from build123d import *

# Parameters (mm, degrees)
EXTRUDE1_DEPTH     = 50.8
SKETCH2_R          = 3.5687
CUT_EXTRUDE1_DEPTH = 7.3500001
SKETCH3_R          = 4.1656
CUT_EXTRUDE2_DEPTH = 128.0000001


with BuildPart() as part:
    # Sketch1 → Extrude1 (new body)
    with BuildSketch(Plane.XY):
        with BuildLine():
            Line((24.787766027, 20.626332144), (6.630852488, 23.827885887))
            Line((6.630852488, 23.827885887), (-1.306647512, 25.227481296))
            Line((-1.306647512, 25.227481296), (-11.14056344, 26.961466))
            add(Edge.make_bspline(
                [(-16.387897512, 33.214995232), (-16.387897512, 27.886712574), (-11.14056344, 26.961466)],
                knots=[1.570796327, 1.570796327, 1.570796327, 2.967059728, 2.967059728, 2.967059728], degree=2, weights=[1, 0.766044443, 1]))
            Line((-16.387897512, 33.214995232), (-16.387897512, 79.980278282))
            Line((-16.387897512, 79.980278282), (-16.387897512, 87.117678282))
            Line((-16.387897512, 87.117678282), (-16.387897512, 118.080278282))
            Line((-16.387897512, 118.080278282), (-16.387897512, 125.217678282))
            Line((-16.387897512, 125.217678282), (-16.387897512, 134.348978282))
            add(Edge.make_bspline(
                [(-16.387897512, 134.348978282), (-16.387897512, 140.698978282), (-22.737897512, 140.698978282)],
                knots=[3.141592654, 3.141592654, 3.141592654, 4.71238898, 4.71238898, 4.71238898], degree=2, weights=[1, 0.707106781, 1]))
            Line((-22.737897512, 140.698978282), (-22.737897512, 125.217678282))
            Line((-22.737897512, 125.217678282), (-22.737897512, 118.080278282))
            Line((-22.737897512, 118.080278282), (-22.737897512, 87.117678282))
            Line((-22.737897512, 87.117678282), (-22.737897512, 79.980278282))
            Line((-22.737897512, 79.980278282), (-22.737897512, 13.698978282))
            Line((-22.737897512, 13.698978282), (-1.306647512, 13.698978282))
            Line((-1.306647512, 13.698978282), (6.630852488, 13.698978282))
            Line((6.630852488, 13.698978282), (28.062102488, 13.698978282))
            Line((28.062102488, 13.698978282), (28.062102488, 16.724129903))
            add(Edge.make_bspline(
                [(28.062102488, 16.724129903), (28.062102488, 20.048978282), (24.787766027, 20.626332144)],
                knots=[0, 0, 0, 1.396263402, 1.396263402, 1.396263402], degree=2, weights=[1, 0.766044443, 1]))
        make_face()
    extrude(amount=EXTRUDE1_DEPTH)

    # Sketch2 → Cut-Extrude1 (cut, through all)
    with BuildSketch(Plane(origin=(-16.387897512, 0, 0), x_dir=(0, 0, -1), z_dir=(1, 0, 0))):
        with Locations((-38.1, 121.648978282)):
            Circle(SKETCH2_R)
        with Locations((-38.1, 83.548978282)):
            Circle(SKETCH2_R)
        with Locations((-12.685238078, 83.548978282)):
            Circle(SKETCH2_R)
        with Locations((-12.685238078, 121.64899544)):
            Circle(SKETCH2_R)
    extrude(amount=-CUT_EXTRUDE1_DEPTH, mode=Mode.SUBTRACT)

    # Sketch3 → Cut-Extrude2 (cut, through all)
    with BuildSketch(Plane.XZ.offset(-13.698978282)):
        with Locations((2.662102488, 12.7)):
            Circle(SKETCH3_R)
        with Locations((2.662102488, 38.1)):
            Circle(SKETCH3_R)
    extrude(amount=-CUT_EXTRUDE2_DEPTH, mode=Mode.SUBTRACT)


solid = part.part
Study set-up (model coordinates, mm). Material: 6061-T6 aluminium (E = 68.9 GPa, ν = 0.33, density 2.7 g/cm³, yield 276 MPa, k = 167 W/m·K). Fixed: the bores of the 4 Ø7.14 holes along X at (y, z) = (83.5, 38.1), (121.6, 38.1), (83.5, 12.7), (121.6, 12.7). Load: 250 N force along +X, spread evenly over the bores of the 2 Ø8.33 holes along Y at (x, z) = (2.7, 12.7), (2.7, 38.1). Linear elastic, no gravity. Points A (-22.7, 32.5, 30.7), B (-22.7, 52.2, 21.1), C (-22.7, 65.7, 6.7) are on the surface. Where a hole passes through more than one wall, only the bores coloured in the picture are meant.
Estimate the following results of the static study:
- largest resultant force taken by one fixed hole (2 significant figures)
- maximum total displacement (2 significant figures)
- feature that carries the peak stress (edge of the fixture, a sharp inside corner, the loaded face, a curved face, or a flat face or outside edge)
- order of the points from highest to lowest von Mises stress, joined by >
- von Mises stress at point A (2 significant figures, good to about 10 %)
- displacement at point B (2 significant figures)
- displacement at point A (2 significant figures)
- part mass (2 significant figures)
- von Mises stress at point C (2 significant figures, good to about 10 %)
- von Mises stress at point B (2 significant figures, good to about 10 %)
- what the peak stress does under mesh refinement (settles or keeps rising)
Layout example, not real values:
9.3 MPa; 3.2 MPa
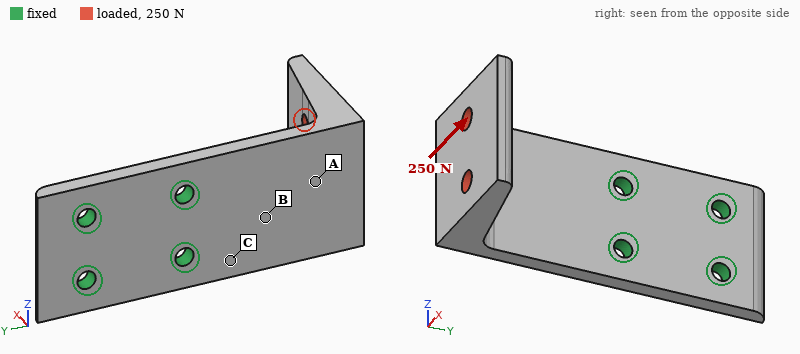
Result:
150 N; 0.43 mm; edge of the fixture; C > B > A; 9.2 MPa; 0.081 mm; 0.19 mm; 170 g; 33 MPa; 22 MPa; keeps rising
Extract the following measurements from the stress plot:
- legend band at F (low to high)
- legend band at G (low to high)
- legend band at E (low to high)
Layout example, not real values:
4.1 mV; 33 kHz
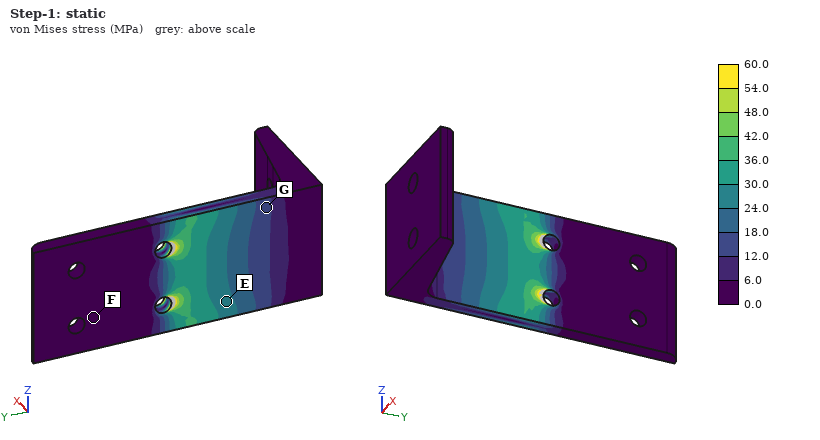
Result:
0.0 to 6.0 MPa; 12.0 to 18.0 MPa; 24.0 to 30.0 MPa
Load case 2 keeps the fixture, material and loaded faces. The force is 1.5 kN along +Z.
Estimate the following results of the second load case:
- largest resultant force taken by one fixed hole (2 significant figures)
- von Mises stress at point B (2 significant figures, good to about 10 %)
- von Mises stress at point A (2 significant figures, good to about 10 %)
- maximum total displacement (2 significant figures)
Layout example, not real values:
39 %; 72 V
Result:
2.9 kN; 61 MPa; 31 MPa; 0.64 mm
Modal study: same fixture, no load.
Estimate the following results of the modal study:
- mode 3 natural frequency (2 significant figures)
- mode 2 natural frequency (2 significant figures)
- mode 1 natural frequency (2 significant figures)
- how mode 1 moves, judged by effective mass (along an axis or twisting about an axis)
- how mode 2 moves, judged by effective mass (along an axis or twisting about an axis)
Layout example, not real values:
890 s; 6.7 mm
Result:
2200 Hz; 1100 Hz; 480 Hz; along X; along Z
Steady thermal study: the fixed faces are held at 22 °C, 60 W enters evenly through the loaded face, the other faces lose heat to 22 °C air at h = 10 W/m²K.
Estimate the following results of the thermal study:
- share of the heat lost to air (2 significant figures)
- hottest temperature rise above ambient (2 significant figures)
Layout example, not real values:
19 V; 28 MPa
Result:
10 %; 73 K
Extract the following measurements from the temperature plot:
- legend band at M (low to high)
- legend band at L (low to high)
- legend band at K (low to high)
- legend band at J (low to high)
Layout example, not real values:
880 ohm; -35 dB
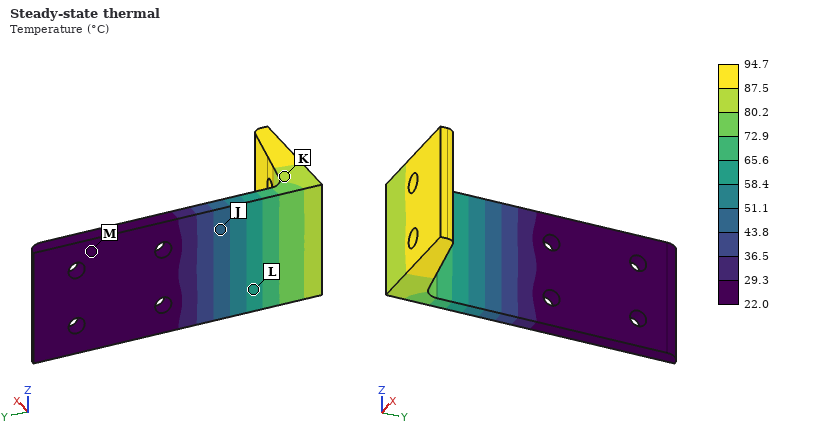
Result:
22.0 to 29.3 °C; 58.4 to 65.6 °C; 80.2 to 87.5 °C; 43.8 to 51.1 °C
